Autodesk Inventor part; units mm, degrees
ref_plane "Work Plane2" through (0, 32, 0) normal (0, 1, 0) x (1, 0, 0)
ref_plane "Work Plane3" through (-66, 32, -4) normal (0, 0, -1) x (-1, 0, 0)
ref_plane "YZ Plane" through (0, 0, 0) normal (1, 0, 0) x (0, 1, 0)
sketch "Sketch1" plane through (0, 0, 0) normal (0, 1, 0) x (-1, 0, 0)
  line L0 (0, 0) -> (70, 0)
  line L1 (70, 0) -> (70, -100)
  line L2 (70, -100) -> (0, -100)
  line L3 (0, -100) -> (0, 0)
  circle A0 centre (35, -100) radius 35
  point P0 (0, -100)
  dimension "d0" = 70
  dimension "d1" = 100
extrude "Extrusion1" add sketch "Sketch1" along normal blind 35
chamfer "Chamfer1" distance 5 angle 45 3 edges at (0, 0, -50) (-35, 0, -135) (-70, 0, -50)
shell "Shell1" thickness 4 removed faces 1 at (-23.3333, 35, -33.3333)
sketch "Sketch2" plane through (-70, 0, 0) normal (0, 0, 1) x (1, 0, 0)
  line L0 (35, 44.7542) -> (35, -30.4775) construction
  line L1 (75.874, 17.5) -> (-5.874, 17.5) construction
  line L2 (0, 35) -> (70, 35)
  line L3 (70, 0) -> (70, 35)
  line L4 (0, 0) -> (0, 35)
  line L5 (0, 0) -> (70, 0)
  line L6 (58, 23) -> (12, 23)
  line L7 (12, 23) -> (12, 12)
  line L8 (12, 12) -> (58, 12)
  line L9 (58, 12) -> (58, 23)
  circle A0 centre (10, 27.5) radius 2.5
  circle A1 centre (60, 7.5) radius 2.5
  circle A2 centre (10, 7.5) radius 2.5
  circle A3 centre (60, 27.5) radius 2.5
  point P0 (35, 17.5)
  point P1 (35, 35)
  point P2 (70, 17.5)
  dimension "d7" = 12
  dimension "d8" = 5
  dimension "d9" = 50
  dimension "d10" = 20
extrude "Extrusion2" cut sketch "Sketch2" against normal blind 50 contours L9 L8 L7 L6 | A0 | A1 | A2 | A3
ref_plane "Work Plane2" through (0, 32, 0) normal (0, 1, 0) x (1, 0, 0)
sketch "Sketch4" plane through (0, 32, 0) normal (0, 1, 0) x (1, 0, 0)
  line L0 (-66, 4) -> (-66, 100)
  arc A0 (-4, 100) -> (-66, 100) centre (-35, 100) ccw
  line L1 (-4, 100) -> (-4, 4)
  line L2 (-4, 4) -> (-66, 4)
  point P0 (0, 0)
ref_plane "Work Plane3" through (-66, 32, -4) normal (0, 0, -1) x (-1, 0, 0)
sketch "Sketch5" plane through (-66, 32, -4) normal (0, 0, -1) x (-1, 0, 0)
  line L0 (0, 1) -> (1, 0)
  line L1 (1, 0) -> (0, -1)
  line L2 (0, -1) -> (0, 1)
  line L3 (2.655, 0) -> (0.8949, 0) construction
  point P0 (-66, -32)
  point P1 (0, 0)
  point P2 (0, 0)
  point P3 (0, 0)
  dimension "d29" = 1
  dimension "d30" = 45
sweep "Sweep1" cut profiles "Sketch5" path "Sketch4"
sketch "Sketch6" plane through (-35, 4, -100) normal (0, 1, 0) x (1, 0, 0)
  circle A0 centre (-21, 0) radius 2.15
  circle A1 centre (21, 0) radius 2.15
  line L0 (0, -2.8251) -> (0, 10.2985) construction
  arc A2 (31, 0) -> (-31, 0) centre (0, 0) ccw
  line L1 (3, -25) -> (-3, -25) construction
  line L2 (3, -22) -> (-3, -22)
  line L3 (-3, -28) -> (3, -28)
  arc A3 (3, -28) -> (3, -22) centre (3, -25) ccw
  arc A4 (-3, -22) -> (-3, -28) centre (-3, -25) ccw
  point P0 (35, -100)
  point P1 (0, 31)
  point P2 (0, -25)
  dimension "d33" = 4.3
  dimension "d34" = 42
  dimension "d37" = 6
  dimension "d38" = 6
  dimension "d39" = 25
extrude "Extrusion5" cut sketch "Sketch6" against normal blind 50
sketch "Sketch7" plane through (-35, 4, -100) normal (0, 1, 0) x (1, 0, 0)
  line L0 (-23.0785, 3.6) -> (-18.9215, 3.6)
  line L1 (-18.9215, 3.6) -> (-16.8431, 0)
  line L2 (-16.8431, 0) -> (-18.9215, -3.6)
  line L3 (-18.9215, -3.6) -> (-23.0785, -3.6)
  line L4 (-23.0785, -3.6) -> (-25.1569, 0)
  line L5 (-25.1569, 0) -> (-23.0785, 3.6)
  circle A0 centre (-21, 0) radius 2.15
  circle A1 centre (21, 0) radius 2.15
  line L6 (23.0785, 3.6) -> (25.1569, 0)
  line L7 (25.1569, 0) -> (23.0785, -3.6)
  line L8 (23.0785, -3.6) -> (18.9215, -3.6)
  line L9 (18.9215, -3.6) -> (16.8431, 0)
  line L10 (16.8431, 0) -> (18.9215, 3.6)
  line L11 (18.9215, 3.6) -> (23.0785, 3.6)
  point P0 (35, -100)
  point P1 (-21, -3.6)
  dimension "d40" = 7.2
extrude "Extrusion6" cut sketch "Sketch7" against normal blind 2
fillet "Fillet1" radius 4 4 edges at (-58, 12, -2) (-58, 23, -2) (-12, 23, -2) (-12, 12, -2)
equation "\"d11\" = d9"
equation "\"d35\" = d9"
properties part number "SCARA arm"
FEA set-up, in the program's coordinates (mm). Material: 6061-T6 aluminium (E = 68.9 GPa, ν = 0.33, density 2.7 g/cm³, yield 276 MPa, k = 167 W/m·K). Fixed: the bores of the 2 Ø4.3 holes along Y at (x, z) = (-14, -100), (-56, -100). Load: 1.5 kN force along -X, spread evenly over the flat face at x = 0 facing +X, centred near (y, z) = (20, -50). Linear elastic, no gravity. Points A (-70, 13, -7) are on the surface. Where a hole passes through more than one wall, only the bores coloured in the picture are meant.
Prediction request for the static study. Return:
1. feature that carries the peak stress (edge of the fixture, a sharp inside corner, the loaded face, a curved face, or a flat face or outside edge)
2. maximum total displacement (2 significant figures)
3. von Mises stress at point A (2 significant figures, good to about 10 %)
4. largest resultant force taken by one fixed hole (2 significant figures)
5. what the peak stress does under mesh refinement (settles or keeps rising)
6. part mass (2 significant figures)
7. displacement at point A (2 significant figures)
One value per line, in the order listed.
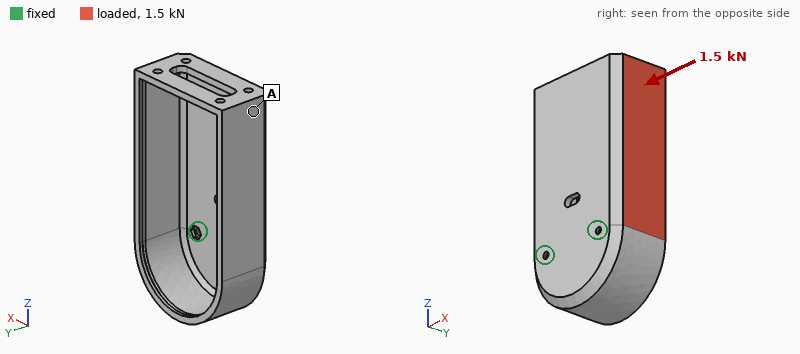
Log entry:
edge of the fixture
0.50 mm
14 MPa
2.1 kN
keeps rising
200 g
0.22 mm
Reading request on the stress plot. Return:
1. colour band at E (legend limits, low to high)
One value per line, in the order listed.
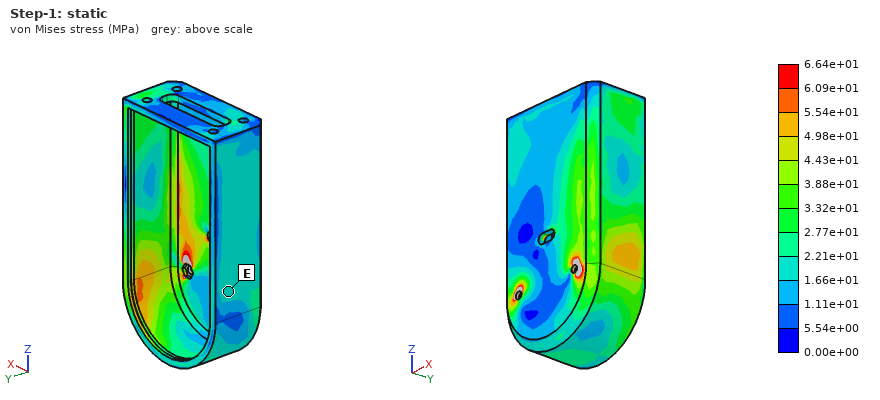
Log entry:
1.66e+01 to 2.21e+01 MPa
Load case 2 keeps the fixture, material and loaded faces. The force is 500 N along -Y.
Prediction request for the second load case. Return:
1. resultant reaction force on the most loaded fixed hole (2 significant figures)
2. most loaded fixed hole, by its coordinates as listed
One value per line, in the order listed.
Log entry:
690 N
(-14, -100)
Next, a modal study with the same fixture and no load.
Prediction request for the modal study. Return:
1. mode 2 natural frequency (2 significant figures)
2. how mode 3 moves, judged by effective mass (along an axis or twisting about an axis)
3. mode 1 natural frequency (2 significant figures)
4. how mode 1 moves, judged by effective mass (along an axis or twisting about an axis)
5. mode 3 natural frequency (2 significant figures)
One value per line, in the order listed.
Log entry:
880 Hz
along X
270 Hz
along Y
2100 Hz
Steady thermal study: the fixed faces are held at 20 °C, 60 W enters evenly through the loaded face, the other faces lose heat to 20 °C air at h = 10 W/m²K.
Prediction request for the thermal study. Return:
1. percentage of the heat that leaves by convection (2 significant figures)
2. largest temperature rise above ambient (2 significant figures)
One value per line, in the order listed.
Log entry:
18 %
61 K
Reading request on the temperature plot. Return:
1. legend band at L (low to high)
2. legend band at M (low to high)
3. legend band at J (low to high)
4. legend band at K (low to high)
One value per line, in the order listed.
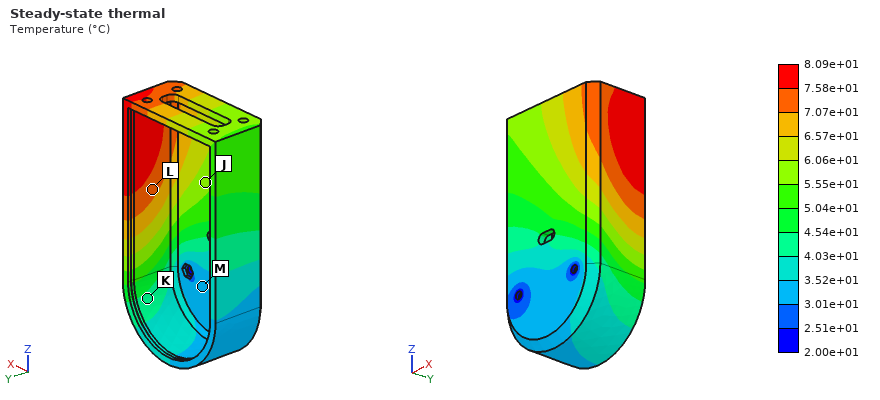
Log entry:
7.07e+01 to 7.58e+01 °C
3.01e+01 to 3.52e+01 °C
5.55e+01 to 6.06e+01 °C
4.03e+01 to 4.54e+01 °C
